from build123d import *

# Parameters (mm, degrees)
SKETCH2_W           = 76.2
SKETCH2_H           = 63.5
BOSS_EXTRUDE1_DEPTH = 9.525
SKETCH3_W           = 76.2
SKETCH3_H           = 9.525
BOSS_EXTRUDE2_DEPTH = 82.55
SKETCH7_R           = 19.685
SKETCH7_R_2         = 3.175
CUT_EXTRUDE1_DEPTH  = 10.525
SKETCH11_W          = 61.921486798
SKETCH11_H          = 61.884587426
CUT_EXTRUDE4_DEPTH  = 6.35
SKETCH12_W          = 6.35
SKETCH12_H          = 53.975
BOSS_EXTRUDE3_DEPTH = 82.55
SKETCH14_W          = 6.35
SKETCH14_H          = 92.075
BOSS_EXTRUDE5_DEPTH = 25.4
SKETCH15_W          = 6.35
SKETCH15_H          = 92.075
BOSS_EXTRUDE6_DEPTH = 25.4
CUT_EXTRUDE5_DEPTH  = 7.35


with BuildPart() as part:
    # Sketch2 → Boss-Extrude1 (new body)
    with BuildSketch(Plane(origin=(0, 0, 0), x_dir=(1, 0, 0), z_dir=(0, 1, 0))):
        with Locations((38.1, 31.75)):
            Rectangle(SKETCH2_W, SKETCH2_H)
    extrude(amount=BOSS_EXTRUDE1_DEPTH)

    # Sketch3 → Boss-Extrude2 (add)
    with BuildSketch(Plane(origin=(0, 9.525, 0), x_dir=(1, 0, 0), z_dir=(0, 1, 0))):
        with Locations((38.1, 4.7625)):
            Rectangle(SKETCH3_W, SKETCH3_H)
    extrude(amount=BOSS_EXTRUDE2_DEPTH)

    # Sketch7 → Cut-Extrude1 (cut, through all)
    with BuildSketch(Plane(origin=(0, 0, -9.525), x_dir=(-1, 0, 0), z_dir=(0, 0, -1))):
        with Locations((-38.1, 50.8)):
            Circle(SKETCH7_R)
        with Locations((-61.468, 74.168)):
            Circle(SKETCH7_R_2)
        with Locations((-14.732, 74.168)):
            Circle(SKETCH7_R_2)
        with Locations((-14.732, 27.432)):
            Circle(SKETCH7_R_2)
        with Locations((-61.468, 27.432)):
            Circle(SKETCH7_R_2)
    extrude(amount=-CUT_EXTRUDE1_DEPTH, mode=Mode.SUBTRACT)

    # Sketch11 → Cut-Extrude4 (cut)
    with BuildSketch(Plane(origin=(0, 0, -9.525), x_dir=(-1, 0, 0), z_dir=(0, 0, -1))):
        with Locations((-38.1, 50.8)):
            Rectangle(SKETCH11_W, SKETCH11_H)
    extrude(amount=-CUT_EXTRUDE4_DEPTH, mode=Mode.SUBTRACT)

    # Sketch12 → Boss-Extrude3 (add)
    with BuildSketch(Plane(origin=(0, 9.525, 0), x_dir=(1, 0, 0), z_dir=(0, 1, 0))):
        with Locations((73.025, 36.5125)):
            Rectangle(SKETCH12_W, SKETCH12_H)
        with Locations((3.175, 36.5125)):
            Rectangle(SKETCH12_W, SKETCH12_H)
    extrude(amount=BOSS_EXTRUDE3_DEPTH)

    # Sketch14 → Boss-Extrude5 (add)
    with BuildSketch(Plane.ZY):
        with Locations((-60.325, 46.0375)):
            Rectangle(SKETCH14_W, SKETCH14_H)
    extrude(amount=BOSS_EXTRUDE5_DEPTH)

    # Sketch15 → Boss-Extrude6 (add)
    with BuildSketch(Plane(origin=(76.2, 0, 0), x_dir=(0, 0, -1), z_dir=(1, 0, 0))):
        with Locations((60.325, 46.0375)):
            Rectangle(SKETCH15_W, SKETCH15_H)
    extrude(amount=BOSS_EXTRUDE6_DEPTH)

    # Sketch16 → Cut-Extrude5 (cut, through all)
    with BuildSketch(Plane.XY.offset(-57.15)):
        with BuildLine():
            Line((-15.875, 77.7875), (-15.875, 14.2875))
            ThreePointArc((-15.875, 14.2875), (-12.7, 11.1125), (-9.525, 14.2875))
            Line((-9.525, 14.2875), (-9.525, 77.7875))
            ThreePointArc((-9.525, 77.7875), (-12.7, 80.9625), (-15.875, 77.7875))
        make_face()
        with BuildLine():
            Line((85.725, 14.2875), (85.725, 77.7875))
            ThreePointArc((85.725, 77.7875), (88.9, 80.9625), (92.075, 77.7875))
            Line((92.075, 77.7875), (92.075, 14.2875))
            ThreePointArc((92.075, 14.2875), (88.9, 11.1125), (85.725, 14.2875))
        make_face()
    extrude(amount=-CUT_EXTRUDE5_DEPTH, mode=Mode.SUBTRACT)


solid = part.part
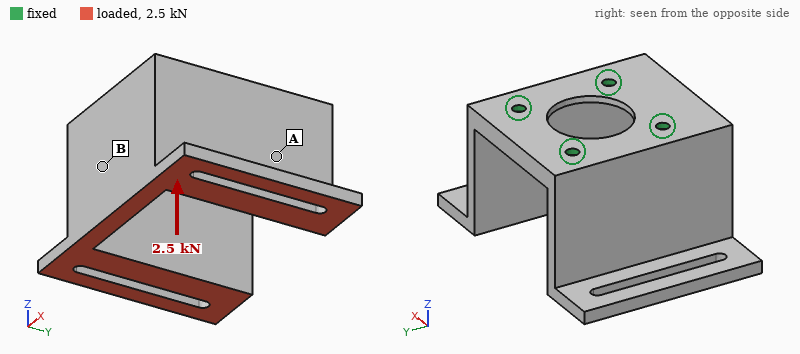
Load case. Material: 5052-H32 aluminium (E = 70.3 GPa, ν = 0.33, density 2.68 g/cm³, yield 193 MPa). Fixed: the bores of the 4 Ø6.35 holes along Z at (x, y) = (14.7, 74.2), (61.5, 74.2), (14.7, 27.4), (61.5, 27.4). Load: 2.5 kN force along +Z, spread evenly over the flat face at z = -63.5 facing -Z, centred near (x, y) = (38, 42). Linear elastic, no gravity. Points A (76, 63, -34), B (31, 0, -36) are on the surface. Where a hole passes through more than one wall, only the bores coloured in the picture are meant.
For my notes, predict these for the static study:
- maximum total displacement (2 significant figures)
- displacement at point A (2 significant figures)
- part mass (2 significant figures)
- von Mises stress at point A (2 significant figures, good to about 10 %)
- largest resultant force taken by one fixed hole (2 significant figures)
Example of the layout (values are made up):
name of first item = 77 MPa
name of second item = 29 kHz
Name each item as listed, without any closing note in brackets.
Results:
maximum total displacement = 0.19 mm
displacement at point A = 0.033 mm
part mass = 420 g
von Mises stress at point A = 11 MPa
largest resultant force taken by one fixed hole = 860 N
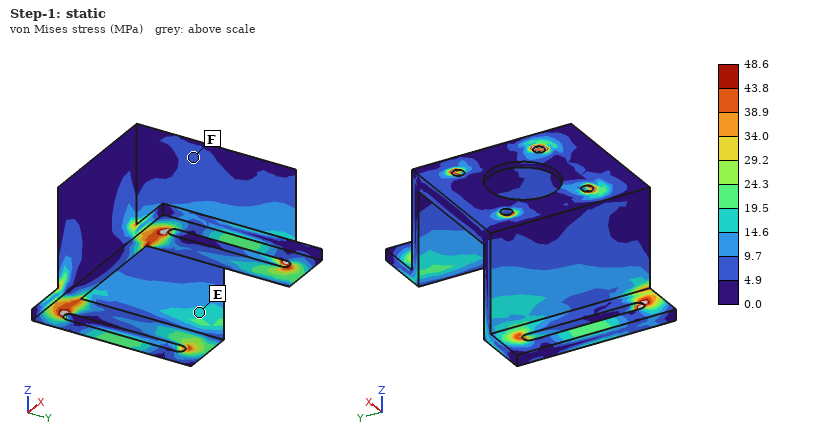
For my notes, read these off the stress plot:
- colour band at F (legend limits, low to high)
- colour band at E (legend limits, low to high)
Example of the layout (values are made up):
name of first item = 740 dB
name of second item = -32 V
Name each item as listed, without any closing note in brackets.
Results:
colour band at F = 4.9 to 9.7 MPa
colour band at E = 14.6 to 19.5 MPa
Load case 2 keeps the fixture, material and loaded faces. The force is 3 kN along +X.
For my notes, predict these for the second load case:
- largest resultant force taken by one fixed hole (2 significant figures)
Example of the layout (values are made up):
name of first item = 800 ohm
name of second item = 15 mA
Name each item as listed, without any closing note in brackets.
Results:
largest resultant force taken by one fixed hole = 4.1 kN
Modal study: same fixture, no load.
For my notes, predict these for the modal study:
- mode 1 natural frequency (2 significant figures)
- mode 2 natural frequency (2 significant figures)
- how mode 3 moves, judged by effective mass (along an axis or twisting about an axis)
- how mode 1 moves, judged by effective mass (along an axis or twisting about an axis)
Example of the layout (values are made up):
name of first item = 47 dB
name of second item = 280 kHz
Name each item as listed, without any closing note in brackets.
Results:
mode 1 natural frequency = 1100 Hz
mode 2 natural frequency = 1200 Hz
how mode 3 moves, judged by effective mass = along Y
how mode 1 moves, judged by effective mass = along X
